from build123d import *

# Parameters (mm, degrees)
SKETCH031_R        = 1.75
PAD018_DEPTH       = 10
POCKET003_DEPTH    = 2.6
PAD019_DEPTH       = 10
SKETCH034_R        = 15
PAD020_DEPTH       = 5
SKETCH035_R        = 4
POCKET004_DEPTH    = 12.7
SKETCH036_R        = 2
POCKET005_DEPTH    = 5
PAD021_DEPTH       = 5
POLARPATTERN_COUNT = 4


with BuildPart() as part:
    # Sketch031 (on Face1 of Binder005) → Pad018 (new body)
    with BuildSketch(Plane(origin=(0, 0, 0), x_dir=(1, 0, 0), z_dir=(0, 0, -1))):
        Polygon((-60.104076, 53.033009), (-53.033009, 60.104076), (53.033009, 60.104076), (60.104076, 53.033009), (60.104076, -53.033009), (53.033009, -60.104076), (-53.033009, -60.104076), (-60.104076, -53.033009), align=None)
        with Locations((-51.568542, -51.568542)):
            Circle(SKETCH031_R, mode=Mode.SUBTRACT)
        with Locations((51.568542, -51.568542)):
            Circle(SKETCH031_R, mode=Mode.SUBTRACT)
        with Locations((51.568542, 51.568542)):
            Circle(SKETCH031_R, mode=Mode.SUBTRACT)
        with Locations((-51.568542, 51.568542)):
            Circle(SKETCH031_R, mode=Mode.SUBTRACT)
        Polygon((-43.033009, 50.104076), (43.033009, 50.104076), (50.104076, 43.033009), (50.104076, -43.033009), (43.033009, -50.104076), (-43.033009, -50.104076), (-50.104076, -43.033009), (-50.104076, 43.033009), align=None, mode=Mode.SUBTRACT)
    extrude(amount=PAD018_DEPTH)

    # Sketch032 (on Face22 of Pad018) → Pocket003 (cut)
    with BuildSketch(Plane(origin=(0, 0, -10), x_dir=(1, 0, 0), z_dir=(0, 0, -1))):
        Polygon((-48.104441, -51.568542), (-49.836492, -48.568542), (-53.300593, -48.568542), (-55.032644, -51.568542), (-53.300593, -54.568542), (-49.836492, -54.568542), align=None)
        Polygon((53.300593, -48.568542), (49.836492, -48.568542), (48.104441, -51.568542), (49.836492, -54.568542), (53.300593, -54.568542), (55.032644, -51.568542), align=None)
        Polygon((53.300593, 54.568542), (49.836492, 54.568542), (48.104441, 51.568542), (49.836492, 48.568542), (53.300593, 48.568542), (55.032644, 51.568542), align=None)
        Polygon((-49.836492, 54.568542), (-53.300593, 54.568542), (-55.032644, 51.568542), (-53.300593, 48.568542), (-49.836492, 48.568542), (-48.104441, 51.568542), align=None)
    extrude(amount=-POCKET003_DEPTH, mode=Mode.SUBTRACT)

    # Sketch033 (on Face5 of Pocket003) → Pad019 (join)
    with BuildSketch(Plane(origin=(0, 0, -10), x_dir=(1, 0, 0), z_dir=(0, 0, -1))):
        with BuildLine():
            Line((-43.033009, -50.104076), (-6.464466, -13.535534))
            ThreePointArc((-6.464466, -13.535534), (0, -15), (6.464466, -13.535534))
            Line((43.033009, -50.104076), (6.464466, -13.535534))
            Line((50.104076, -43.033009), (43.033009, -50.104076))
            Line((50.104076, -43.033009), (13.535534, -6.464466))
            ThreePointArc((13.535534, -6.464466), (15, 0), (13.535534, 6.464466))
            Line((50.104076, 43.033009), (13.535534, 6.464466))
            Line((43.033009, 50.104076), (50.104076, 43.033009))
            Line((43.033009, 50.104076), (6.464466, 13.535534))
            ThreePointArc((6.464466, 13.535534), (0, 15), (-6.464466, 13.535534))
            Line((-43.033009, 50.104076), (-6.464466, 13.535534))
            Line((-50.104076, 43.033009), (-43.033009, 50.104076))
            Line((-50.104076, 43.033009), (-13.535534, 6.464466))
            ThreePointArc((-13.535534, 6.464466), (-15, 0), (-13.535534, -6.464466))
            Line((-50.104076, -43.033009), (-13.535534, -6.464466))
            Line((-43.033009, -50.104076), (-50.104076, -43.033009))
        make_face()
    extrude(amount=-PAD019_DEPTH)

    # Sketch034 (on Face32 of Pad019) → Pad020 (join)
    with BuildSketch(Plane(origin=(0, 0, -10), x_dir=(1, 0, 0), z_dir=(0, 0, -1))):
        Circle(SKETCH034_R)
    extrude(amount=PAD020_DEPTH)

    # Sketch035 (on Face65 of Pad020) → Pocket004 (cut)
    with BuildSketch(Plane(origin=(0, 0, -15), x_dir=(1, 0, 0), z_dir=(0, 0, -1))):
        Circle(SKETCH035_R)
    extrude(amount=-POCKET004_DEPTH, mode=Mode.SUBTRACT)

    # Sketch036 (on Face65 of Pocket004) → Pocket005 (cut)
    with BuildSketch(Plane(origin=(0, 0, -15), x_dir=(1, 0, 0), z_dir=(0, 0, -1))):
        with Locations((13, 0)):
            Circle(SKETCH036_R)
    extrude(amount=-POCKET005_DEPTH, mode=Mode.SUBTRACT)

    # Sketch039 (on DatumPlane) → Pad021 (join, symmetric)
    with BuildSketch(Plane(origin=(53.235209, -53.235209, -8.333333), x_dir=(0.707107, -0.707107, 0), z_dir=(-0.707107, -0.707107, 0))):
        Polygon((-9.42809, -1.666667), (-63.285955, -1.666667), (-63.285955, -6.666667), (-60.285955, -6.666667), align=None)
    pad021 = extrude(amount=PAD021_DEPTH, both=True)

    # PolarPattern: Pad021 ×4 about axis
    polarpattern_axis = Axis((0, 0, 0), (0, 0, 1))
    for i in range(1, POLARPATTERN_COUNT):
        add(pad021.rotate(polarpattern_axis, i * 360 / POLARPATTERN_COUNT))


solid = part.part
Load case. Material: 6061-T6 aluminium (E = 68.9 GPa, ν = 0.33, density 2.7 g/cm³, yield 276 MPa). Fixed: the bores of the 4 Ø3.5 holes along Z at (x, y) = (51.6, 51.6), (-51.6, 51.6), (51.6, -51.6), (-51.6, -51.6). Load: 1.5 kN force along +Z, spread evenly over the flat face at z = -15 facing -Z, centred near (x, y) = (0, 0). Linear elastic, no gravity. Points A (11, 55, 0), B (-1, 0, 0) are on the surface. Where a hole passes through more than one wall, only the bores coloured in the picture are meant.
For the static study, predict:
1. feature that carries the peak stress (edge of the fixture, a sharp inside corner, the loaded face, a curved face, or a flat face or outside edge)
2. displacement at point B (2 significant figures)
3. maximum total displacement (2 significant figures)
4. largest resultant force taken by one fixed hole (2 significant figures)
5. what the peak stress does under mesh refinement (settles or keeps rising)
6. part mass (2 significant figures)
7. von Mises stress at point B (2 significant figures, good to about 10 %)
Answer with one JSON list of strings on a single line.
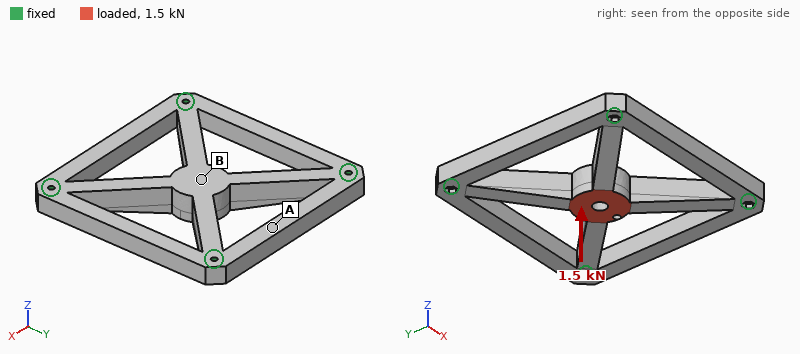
["a sharp inside corner", "87 µm", "88 µm", "720 N", "keeps rising", "210 g", "16 MPa"]
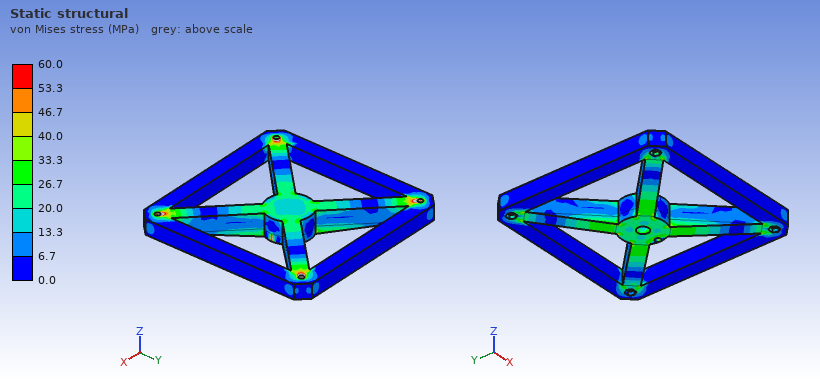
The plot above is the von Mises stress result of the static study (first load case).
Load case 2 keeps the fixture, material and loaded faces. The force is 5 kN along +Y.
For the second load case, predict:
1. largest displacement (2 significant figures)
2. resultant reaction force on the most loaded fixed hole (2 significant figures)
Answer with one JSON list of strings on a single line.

["37 µm", "1.7 kN"]
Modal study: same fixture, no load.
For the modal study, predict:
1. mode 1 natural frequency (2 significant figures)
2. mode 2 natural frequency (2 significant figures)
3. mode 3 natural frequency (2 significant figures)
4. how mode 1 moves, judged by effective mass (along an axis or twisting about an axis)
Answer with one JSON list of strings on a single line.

["2700 Hz", "4100 Hz", "4300 Hz", "along Z"]
